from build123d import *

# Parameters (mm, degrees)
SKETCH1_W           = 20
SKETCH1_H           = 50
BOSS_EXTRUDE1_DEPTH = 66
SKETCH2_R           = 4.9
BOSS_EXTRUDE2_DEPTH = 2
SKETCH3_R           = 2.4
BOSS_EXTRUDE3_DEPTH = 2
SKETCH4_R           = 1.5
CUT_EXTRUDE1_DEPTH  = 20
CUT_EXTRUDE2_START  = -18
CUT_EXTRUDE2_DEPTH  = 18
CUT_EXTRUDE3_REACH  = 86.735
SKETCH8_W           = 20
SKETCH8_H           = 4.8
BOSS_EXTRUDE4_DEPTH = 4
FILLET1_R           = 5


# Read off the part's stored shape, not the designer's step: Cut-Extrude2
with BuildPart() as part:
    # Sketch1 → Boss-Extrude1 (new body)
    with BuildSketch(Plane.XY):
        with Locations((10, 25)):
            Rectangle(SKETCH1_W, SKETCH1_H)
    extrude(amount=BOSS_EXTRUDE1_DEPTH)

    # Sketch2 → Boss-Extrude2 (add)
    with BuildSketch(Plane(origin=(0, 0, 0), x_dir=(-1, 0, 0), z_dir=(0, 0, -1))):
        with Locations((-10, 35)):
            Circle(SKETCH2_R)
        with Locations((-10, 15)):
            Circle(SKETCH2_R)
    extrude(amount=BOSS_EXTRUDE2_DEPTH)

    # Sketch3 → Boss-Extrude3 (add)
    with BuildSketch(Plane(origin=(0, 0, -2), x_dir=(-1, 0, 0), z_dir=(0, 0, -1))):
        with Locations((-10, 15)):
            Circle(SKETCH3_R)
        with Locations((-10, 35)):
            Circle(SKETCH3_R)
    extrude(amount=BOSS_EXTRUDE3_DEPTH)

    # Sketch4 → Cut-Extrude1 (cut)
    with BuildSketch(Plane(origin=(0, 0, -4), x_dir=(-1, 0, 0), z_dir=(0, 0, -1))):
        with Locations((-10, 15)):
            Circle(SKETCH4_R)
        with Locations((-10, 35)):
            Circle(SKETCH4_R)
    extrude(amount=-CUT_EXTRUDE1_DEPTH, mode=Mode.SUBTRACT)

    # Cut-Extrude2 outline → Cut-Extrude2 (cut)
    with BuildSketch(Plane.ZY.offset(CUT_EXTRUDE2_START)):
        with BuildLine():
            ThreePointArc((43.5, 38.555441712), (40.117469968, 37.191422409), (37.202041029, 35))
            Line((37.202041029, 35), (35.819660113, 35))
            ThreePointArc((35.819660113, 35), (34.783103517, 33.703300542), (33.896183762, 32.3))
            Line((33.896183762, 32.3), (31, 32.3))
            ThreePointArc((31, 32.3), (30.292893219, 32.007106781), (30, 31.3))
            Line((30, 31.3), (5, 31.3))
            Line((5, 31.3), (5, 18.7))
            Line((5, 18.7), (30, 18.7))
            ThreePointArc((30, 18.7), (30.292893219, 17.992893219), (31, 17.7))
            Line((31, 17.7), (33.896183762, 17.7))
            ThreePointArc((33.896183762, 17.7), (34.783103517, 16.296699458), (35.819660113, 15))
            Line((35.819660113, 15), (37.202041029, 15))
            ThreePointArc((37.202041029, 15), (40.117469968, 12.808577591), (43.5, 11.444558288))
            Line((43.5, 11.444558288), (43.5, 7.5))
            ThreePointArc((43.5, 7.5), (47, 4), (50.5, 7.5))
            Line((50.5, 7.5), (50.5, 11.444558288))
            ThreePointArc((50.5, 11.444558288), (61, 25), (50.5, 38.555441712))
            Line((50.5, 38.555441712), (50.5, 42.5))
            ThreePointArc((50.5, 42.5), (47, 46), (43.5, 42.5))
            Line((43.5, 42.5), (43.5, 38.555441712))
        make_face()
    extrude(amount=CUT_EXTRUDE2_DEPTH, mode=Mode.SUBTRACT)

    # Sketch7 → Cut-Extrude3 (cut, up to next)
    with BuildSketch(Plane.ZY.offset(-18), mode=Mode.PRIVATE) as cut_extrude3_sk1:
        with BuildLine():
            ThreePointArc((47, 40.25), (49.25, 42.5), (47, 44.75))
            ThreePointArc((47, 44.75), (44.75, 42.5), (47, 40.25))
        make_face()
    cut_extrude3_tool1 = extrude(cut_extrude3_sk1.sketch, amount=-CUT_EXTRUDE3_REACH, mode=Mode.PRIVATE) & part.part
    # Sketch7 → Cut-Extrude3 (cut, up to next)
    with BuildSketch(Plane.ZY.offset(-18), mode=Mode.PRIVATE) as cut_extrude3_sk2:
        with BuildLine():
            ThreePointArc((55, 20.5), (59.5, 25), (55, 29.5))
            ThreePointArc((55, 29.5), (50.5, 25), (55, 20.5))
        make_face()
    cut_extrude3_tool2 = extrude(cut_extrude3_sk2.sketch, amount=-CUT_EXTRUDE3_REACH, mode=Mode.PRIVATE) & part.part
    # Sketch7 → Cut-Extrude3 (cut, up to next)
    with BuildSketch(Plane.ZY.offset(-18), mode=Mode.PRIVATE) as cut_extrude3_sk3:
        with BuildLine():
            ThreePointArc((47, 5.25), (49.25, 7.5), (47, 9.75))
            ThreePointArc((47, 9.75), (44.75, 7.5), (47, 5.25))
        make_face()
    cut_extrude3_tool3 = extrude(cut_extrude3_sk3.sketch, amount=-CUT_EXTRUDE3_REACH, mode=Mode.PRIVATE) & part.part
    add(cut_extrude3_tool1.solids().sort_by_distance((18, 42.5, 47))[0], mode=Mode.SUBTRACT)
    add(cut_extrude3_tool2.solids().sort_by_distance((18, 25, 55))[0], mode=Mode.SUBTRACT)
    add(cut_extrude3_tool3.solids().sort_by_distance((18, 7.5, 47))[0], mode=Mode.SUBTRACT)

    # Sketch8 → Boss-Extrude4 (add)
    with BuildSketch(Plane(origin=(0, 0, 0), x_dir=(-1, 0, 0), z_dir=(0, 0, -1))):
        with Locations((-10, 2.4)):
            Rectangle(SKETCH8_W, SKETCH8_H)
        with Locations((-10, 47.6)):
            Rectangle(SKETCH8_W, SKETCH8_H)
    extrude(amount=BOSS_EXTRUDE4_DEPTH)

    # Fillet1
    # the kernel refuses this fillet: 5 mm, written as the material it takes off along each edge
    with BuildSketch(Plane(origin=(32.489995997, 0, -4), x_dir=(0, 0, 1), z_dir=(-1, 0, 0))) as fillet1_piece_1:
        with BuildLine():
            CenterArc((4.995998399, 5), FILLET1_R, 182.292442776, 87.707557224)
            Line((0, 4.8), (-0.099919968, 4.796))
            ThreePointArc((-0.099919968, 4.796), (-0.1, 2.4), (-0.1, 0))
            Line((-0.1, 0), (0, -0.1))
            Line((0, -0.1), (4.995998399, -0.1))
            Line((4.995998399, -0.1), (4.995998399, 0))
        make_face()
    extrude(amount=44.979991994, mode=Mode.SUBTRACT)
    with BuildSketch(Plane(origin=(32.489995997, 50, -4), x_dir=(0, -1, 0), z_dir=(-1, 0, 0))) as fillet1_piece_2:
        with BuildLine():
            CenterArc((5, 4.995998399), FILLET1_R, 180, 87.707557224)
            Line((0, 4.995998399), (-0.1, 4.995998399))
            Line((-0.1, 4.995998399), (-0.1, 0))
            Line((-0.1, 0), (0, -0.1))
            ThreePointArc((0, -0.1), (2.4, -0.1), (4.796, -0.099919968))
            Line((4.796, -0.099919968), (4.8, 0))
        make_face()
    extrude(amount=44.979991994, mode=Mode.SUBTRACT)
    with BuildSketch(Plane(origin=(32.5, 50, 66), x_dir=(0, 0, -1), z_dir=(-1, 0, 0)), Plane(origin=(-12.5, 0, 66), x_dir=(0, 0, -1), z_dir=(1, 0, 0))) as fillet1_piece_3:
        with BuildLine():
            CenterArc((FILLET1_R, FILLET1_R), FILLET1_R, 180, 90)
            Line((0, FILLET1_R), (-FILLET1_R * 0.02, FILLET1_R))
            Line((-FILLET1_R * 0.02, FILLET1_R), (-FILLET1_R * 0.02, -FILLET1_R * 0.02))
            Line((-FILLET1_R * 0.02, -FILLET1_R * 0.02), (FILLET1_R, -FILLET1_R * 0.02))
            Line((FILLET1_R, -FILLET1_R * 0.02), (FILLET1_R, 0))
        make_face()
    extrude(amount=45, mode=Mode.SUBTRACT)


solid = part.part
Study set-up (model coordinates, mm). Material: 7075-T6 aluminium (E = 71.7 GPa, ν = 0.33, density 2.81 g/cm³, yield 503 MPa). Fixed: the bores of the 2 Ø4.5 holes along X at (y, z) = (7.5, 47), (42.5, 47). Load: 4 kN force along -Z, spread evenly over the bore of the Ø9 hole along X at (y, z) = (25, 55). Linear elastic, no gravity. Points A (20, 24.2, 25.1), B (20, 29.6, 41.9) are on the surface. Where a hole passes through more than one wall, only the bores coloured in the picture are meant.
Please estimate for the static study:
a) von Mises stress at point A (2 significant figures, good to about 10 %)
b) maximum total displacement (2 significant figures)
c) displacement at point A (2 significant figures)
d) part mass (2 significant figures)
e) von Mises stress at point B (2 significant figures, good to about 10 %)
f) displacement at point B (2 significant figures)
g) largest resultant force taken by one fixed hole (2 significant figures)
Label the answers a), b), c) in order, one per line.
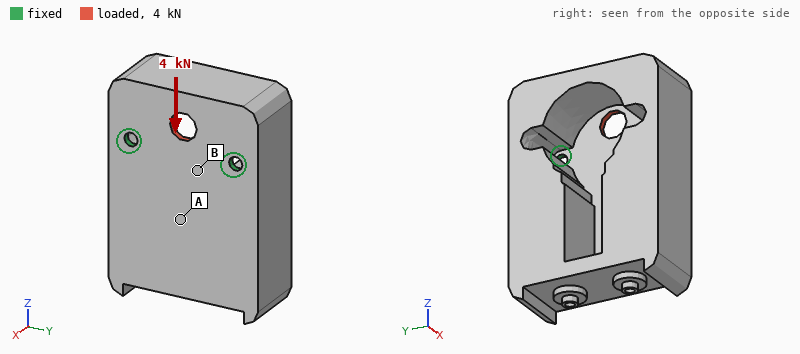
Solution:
a) 14 MPa
b) 26 µm
c) 5.2 µm
d) 130 g
e) 36 MPa
f) 9.3 µm
g) 2.1 kN
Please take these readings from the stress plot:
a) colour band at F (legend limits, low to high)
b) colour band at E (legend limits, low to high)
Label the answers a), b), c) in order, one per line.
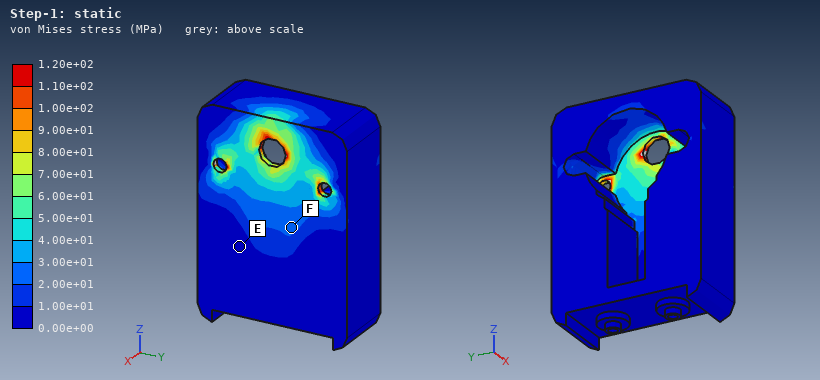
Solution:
a) 2.00e+01 to 3.00e+01 MPa
b) 0.00e+00 to 1.00e+01 MPa
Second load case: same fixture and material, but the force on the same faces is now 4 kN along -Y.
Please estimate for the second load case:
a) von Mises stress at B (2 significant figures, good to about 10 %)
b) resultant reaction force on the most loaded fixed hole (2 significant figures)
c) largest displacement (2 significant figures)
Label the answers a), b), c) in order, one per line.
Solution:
a) 20 MPa
b) 2.2 kN
c) 22 µm
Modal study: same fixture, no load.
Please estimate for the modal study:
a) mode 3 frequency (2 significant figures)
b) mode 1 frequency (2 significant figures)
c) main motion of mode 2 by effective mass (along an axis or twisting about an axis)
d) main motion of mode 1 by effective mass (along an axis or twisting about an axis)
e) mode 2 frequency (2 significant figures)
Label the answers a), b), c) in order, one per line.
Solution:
a) 5500 Hz
b) 850 Hz
c) along Y
d) along X
e) 3800 Hz
